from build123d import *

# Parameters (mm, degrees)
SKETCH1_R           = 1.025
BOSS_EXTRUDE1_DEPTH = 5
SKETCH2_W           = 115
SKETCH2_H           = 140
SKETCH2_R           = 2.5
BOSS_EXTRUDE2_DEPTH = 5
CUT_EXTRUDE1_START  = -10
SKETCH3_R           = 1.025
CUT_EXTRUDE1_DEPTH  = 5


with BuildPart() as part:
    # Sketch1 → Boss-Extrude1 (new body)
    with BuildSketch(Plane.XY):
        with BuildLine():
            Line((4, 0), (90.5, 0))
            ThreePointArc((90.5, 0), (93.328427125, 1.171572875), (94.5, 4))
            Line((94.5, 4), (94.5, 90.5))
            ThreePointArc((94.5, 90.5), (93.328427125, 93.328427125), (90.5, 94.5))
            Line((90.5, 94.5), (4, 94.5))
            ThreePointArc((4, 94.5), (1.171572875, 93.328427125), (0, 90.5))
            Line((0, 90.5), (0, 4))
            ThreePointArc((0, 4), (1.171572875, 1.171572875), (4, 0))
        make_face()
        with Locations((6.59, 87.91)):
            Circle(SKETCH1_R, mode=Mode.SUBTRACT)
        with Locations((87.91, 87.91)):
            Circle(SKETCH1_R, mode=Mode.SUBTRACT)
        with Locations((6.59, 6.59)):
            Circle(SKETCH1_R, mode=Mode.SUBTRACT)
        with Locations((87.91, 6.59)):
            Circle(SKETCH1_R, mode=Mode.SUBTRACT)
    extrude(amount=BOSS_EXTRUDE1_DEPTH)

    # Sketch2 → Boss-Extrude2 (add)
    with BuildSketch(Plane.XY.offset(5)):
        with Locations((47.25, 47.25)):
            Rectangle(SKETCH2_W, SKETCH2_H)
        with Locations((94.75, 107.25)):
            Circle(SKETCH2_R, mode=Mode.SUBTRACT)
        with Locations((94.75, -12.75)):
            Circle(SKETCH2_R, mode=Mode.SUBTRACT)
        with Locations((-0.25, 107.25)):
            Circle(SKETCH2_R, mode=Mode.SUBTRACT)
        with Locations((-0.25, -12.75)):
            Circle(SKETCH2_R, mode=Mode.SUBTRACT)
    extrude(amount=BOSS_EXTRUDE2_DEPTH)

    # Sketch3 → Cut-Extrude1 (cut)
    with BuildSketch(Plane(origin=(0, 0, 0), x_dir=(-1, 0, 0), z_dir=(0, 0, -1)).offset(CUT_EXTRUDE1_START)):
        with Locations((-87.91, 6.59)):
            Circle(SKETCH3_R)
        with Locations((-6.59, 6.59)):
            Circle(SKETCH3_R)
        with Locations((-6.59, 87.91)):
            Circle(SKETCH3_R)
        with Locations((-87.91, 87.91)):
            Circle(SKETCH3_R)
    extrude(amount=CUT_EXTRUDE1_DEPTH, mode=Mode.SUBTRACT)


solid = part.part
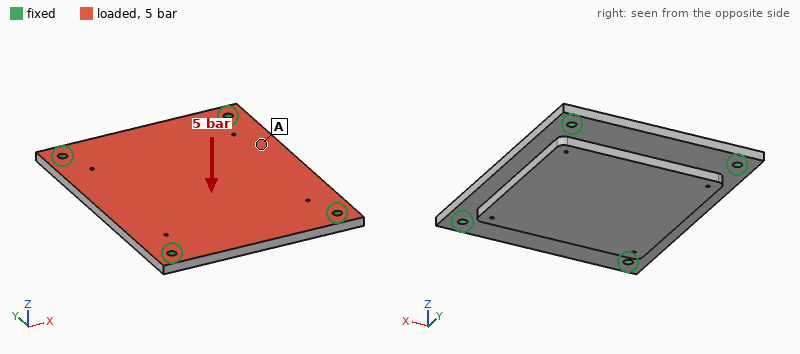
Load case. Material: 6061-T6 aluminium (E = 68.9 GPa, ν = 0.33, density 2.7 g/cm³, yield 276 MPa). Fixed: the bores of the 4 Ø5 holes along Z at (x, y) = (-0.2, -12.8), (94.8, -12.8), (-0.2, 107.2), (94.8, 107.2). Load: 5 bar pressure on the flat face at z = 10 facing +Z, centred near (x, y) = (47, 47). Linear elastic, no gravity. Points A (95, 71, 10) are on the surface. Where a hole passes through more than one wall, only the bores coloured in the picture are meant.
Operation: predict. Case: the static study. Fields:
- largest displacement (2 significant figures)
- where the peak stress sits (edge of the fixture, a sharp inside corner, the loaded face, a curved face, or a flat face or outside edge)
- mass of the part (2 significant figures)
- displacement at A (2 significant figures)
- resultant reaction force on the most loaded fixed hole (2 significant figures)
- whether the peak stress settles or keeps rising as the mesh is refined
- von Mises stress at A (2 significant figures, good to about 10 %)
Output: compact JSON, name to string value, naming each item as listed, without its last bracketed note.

{"largest displacement": "0.20 mm", "where the peak stress sits": "edge of the fixture", "mass of the part": "340 g", "displacement at A": "0.14 mm", "resultant reaction force on the most loaded fixed hole": "3.0 kN", "whether the peak stress settles or keeps rising as the mesh is refined": "keeps rising", "von Mises stress at A": "27 MPa"}
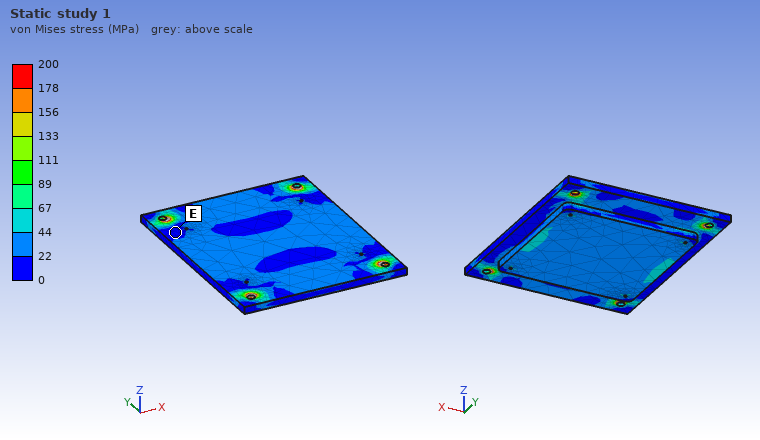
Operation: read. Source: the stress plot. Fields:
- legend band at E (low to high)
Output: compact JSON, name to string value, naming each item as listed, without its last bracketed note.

{"legend band at E": "0 to 22 MPa"}
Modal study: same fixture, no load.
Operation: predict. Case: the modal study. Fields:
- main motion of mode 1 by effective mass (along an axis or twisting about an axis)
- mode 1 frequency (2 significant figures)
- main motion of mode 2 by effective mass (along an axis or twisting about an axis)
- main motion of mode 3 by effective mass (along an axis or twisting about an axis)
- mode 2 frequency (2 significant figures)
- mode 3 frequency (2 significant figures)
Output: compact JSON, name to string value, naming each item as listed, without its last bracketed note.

{"main motion of mode 1 by effective mass": "along Z", "mode 1 frequency": "1800 Hz", "main motion of mode 2 by effective mass": "twisting about Y", "main motion of mode 3 by effective mass": "twisting about X", "mode 2 frequency": "2900 Hz", "mode 3 frequency": "3500 Hz"}
